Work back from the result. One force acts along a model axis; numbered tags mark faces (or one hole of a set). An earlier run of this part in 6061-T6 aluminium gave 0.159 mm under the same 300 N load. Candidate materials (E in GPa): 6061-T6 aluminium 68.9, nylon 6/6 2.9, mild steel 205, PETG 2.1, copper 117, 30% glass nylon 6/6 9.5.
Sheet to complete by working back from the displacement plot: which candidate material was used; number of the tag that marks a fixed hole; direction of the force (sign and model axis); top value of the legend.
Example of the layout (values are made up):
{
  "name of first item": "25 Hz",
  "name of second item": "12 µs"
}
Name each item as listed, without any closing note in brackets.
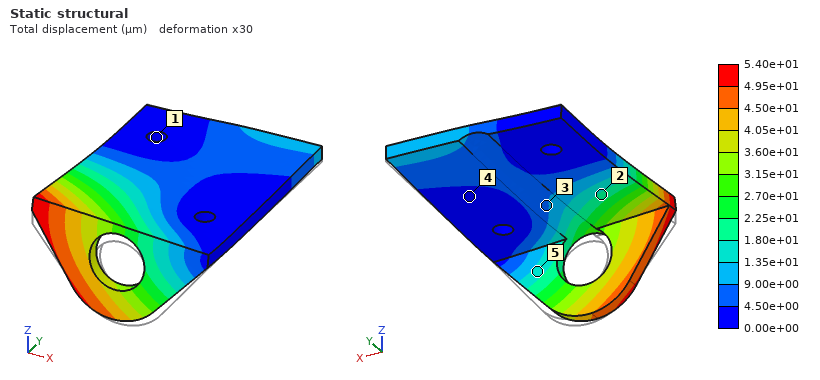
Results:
{
  "which candidate material was used": "mild steel",
  "number of the tag that marks a fixed hole": "1",
  "direction of the force": "+Z",
  "top value of the legend": "5.40e+01 µm"
}
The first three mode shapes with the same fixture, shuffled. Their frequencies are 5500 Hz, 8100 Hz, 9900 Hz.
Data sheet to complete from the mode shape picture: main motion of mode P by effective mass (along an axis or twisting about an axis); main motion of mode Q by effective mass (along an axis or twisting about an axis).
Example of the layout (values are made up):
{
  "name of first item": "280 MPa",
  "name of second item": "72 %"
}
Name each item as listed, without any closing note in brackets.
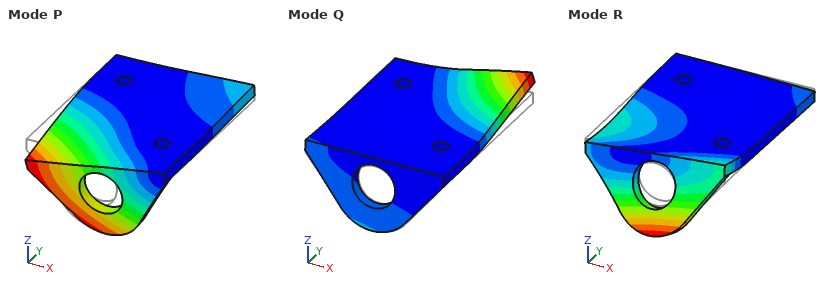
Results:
{
  "main motion of mode P by effective mass": "along Z",
  "main motion of mode Q by effective mass": "along Z"
}
